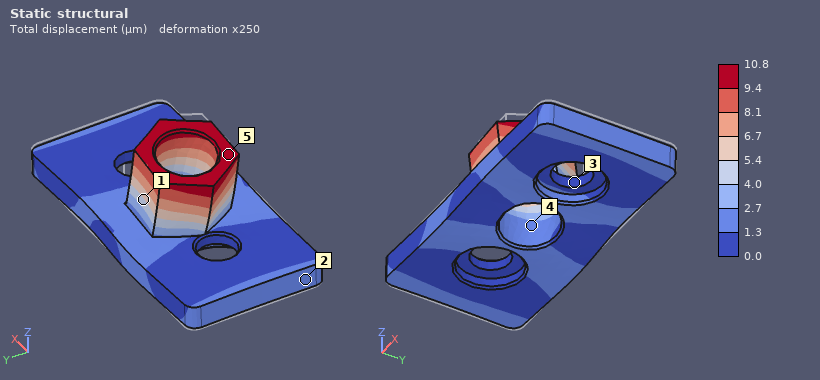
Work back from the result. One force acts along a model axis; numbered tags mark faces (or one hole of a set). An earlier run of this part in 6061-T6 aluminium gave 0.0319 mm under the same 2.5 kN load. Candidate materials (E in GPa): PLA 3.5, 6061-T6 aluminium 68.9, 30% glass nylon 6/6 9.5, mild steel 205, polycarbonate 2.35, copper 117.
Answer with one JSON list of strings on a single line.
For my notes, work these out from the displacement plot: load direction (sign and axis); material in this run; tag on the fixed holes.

["-X", "mild steel", "3"]
